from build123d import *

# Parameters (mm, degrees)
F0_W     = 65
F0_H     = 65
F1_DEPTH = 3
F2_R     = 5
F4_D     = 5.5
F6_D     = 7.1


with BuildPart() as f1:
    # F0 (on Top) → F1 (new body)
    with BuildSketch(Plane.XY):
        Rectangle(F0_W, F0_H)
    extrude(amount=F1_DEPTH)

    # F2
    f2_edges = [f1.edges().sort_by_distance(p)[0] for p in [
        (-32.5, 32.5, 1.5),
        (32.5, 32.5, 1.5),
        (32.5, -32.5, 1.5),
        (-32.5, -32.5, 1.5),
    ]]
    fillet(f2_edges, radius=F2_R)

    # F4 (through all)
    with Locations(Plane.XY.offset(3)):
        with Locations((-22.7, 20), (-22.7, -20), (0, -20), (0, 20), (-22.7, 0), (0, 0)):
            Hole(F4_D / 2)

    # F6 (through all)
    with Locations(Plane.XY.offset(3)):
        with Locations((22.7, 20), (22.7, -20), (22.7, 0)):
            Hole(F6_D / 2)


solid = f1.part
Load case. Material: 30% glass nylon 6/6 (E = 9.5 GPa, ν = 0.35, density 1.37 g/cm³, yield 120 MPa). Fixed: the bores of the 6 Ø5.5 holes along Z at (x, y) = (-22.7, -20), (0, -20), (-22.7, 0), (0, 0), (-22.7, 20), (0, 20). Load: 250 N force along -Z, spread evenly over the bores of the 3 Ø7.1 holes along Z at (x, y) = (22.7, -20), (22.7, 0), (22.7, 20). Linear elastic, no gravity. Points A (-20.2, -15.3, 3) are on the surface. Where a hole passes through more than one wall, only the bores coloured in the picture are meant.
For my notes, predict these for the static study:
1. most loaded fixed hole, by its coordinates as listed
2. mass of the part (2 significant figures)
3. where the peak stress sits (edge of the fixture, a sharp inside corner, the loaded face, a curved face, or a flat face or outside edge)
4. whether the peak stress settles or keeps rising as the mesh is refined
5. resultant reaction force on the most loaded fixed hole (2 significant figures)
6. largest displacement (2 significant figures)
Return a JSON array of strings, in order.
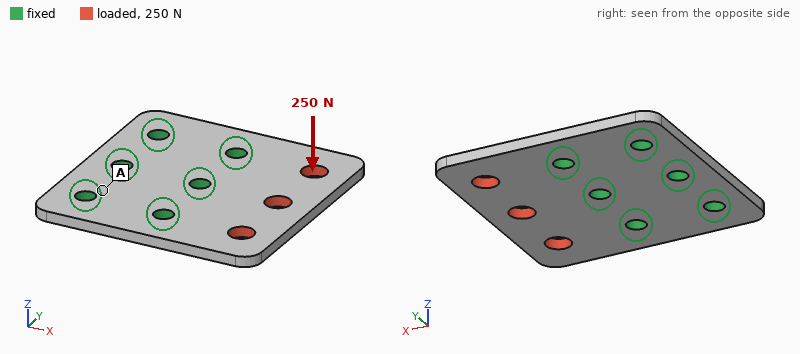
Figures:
["(0, 0)", "16 g", "edge of the fixture", "keeps rising", "100 N", "1.0 mm"]
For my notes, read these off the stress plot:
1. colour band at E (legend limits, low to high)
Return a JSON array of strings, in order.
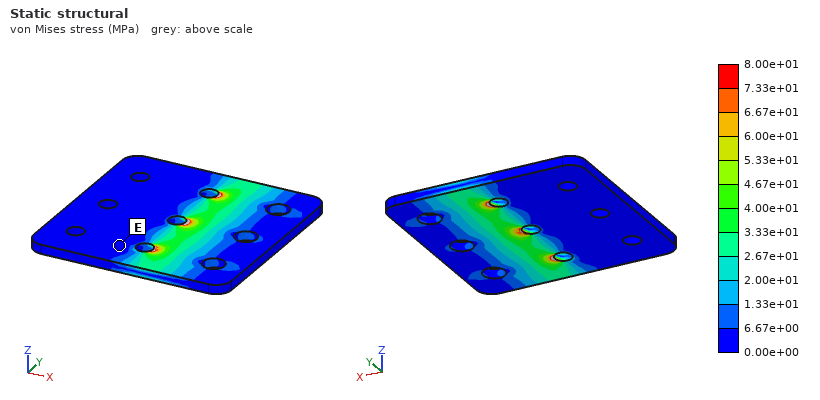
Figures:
["0.00e+00 to 6.67e+00 MPa"]
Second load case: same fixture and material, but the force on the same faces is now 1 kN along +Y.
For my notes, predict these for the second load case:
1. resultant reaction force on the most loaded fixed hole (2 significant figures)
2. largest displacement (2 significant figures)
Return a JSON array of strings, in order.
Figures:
["510 N", "68 µm"]
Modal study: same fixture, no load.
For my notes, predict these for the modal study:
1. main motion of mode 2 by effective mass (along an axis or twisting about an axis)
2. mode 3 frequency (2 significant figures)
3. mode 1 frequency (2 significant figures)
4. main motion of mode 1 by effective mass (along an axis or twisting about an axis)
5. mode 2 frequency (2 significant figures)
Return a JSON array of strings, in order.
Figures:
["twisting about X", "3400 Hz", "1400 Hz", "along Z", "1900 Hz"]
